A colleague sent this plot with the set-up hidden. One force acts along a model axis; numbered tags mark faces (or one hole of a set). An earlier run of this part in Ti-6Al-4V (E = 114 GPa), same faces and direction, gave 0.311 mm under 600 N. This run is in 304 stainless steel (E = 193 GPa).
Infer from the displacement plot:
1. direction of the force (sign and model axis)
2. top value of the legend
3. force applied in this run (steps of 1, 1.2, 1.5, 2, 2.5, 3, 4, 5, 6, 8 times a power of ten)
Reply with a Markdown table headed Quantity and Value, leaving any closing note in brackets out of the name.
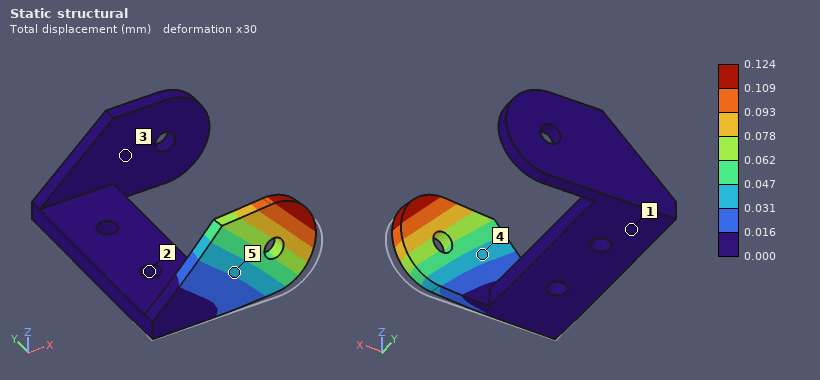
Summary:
| Quantity | Value |
|---|---|
| direction of the force | +Y |
| top value of the legend | 0.124 mm |
| force applied in this run | 400 N |
